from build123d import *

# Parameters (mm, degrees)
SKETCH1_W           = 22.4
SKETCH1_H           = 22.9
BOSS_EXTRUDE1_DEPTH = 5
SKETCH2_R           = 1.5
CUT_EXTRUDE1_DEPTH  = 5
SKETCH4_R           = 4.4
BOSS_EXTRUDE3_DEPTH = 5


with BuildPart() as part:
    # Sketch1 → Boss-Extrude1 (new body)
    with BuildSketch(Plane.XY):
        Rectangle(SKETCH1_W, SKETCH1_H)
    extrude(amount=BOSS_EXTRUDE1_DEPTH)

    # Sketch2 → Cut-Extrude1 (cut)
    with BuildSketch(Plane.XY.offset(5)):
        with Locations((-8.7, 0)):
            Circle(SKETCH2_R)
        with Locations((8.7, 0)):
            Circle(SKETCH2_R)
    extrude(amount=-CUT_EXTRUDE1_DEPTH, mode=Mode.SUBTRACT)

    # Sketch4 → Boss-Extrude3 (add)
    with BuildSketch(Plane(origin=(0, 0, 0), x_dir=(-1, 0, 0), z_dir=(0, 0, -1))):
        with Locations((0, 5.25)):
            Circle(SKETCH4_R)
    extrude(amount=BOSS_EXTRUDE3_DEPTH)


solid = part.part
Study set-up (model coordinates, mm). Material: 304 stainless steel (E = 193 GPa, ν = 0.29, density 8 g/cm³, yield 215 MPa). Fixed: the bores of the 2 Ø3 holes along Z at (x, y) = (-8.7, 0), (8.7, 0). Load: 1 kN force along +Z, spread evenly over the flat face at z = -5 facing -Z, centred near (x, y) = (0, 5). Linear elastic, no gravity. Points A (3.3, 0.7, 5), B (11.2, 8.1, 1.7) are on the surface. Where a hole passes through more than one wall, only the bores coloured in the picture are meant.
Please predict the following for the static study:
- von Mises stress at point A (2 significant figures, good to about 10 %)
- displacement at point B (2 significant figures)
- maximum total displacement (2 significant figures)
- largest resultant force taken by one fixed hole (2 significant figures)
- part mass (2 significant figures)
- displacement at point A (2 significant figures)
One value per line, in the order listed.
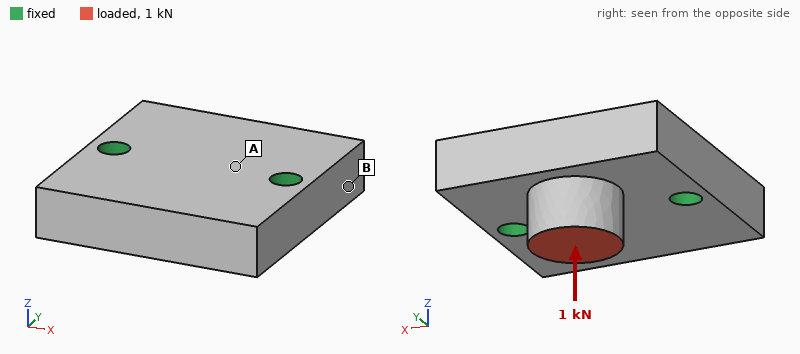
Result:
22 MPa
2.4 µm
6.9 µm
500 N
22 g
1.4 µm
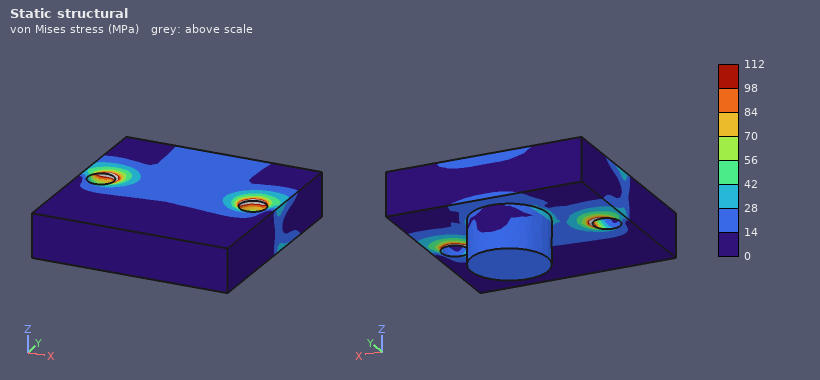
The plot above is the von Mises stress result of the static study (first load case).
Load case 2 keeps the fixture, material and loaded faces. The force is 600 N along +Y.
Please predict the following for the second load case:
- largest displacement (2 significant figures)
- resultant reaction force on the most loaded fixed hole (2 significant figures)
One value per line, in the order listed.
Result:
8.3 µm
310 N
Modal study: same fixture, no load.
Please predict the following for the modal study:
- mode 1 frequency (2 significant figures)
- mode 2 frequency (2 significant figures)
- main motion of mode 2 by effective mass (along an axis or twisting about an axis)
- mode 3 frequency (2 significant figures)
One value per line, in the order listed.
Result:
20 kHz
27 kHz
along Z
40 kHz
